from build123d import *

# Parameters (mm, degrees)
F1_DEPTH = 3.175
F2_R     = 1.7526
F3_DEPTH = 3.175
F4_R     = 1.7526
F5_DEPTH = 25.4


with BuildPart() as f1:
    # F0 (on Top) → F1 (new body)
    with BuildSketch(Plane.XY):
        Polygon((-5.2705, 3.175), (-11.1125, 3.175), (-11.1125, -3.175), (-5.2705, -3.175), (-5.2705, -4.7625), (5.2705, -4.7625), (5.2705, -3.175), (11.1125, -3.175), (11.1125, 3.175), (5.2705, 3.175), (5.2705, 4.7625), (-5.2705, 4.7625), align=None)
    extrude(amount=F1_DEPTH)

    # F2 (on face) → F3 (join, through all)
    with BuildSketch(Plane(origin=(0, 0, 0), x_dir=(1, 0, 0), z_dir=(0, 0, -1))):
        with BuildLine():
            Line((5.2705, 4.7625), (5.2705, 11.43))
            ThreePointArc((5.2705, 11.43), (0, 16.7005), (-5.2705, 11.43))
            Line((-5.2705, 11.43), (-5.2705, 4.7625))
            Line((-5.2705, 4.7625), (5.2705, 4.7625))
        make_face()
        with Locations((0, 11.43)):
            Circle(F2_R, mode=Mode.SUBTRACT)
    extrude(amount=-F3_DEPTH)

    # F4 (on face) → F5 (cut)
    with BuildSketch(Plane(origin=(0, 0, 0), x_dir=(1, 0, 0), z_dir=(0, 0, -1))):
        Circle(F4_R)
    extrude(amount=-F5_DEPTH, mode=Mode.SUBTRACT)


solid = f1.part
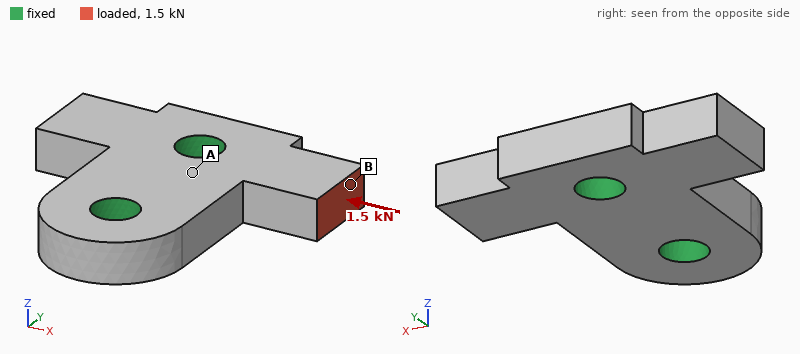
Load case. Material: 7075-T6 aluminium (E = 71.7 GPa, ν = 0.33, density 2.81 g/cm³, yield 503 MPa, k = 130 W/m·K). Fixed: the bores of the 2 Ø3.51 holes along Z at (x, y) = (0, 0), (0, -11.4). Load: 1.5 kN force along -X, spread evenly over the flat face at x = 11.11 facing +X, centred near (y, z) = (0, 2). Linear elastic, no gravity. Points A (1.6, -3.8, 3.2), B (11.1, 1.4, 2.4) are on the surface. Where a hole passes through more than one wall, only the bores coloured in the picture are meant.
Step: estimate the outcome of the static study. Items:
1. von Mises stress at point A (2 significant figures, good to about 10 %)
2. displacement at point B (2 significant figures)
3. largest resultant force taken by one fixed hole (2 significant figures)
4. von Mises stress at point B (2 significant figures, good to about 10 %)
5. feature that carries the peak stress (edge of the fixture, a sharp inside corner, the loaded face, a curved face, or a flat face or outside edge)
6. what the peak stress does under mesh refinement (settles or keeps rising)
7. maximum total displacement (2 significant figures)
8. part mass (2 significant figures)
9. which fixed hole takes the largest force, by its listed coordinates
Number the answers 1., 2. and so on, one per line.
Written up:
1. 18 MPa
2. 11 µm
3. 1.4 kN
4. 74 MPa
5. edge of the fixture
6. keeps rising
7. 11 µm
8. 2.4 g
9. (0, 0)
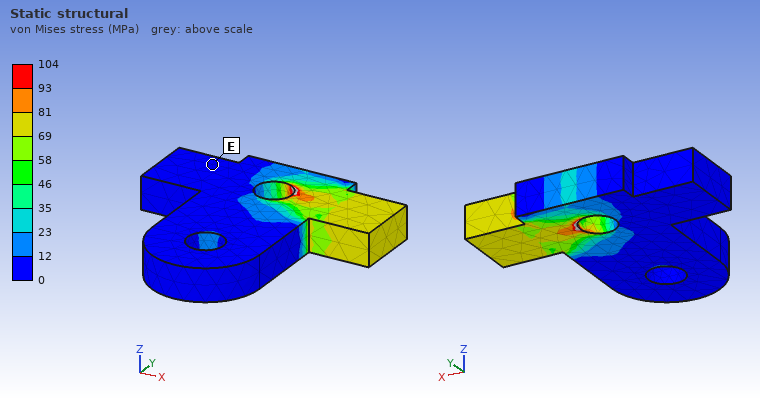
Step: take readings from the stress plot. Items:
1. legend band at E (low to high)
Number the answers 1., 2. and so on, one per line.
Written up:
1. 0 to 12 MPa
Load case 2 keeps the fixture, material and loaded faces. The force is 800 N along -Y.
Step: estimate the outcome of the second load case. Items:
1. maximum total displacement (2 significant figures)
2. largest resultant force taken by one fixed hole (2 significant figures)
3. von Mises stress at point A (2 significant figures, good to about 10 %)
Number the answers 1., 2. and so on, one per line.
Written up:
1. 52 µm
2. 640 N
3. 56 MPa
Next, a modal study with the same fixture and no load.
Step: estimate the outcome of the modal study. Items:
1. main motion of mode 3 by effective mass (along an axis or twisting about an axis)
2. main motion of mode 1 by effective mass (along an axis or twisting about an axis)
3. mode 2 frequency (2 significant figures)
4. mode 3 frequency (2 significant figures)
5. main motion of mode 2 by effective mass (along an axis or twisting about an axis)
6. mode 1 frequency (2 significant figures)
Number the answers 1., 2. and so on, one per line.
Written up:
1. twisting about Z
2. twisting about Y
3. 28 kHz
4. 49 kHz
5. along Z
6. 27 kHz
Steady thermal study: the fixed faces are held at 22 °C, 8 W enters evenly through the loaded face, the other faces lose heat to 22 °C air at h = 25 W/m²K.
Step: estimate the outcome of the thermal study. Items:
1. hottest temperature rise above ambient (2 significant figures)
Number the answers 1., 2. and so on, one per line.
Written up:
1. 27 K
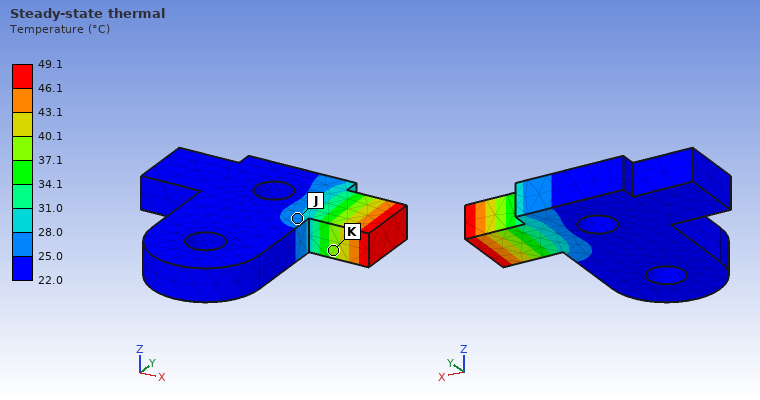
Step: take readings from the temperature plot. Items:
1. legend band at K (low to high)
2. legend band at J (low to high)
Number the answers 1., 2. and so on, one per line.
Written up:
1. 37.1 to 40.1 °C
2. 25.0 to 28.0 °C
